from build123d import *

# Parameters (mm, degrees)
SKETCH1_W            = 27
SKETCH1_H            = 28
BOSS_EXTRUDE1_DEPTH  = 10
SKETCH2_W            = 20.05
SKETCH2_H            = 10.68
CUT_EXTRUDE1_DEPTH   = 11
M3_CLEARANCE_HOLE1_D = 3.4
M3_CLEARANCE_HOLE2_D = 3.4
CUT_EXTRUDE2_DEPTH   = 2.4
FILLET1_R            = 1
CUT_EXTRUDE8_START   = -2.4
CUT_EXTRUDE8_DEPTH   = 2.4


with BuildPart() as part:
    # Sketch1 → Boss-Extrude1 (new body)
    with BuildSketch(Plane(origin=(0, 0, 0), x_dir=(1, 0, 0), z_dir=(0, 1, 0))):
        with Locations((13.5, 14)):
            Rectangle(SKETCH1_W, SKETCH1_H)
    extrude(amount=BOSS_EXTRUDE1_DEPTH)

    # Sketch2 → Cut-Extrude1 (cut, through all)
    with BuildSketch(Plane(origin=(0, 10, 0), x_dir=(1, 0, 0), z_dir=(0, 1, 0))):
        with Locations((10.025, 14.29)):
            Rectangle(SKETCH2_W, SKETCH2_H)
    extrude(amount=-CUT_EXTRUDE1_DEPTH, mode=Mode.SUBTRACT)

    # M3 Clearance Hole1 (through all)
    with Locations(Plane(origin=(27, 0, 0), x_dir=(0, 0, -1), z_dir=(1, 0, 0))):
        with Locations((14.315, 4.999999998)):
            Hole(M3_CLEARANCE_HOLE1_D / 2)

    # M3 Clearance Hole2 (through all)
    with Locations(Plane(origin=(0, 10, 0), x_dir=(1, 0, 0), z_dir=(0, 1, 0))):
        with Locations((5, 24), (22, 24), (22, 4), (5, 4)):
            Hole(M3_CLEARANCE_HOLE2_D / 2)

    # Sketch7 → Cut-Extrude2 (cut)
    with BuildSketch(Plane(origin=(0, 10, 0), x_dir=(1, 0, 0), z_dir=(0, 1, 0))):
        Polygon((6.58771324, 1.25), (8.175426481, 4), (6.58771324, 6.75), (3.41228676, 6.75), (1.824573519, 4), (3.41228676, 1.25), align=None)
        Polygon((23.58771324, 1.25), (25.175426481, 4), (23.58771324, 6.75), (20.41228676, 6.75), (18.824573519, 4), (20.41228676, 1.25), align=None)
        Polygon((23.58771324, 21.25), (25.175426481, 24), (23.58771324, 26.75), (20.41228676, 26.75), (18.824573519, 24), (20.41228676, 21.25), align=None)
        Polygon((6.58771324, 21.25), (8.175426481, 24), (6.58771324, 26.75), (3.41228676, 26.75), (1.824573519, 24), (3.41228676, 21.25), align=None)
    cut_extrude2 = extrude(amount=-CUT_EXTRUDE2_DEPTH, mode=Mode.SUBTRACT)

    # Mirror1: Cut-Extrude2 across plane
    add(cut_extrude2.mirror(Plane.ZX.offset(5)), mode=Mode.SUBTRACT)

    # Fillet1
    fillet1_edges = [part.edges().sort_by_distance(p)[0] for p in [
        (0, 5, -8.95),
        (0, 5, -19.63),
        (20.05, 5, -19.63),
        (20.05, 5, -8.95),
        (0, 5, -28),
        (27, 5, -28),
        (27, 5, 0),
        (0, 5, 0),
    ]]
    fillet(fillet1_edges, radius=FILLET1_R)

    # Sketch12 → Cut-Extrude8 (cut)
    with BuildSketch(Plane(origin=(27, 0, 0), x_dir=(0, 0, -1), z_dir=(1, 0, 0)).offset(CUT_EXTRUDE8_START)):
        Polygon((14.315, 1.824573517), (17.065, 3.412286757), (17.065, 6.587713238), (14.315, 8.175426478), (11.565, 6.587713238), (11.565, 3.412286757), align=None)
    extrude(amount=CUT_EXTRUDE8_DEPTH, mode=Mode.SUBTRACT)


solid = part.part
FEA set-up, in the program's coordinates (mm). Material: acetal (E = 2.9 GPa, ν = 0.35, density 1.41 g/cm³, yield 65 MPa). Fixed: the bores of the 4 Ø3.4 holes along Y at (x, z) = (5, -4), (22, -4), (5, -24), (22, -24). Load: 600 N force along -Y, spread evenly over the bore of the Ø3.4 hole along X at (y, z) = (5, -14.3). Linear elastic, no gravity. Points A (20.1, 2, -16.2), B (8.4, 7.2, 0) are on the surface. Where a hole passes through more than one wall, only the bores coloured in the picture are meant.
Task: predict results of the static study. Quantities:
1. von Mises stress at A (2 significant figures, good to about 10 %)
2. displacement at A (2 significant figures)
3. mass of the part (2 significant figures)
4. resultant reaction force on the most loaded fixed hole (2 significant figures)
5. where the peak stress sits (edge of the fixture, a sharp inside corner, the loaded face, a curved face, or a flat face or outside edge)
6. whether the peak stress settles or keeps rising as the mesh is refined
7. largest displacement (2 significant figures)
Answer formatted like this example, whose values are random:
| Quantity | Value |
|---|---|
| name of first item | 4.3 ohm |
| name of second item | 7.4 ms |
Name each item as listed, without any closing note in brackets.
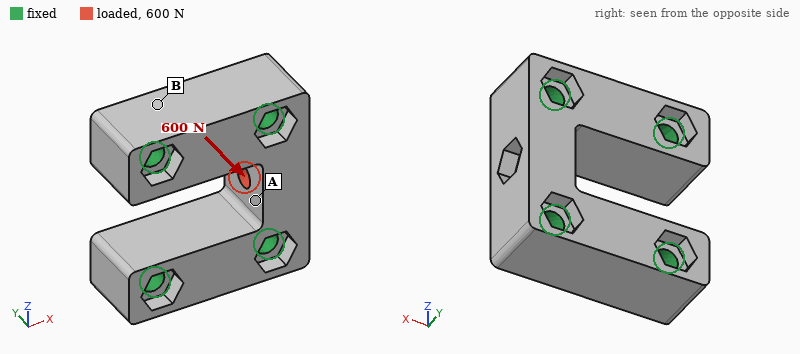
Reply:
| Quantity | Value |
|---|---|
| von Mises stress at A | 14 MPa |
| displacement at A | 64 µm |
| mass of the part | 6.5 g |
| resultant reaction force on the most loaded fixed hole | 300 N |
| where the peak stress sits | edge of the fixture |
| whether the peak stress settles or keeps rising as the mesh is refined | keeps rising |
| largest displacement | 79 µm |
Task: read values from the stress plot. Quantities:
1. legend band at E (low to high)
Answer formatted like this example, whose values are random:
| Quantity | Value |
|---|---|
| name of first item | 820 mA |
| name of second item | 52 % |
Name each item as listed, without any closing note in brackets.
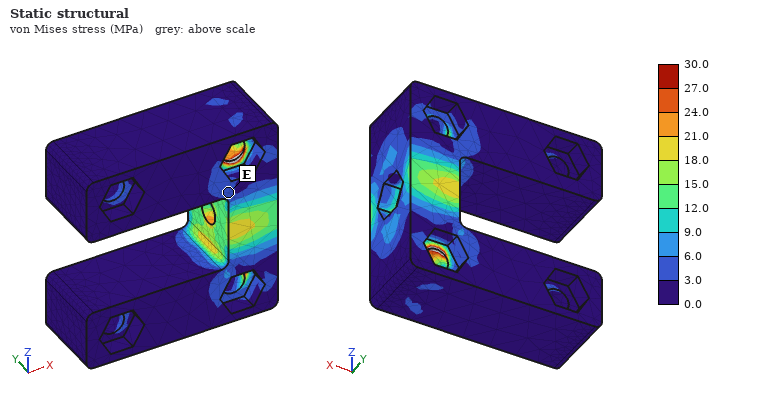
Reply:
| Quantity | Value |
|---|---|
| legend band at E | 3.0 to 6.0 MPa |
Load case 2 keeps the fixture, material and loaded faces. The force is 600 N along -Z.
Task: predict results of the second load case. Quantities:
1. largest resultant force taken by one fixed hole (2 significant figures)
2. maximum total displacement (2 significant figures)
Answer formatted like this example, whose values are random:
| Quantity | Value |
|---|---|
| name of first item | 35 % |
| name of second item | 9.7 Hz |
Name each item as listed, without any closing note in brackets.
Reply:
| Quantity | Value |
|---|---|
| largest resultant force taken by one fixed hole | 300 N |
| maximum total displacement | 27 µm |
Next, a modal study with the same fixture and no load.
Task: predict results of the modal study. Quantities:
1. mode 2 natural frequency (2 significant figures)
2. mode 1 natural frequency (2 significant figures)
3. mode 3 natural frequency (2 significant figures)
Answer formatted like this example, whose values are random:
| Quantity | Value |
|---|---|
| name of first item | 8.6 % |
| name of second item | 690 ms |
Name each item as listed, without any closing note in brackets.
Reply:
| Quantity | Value |
|---|---|
| mode 2 natural frequency | 16 kHz |
| mode 1 natural frequency | 15 kHz |
| mode 3 natural frequency | 17 kHz |
